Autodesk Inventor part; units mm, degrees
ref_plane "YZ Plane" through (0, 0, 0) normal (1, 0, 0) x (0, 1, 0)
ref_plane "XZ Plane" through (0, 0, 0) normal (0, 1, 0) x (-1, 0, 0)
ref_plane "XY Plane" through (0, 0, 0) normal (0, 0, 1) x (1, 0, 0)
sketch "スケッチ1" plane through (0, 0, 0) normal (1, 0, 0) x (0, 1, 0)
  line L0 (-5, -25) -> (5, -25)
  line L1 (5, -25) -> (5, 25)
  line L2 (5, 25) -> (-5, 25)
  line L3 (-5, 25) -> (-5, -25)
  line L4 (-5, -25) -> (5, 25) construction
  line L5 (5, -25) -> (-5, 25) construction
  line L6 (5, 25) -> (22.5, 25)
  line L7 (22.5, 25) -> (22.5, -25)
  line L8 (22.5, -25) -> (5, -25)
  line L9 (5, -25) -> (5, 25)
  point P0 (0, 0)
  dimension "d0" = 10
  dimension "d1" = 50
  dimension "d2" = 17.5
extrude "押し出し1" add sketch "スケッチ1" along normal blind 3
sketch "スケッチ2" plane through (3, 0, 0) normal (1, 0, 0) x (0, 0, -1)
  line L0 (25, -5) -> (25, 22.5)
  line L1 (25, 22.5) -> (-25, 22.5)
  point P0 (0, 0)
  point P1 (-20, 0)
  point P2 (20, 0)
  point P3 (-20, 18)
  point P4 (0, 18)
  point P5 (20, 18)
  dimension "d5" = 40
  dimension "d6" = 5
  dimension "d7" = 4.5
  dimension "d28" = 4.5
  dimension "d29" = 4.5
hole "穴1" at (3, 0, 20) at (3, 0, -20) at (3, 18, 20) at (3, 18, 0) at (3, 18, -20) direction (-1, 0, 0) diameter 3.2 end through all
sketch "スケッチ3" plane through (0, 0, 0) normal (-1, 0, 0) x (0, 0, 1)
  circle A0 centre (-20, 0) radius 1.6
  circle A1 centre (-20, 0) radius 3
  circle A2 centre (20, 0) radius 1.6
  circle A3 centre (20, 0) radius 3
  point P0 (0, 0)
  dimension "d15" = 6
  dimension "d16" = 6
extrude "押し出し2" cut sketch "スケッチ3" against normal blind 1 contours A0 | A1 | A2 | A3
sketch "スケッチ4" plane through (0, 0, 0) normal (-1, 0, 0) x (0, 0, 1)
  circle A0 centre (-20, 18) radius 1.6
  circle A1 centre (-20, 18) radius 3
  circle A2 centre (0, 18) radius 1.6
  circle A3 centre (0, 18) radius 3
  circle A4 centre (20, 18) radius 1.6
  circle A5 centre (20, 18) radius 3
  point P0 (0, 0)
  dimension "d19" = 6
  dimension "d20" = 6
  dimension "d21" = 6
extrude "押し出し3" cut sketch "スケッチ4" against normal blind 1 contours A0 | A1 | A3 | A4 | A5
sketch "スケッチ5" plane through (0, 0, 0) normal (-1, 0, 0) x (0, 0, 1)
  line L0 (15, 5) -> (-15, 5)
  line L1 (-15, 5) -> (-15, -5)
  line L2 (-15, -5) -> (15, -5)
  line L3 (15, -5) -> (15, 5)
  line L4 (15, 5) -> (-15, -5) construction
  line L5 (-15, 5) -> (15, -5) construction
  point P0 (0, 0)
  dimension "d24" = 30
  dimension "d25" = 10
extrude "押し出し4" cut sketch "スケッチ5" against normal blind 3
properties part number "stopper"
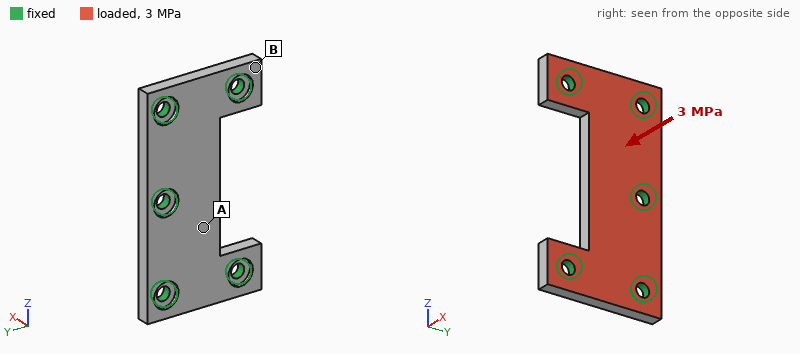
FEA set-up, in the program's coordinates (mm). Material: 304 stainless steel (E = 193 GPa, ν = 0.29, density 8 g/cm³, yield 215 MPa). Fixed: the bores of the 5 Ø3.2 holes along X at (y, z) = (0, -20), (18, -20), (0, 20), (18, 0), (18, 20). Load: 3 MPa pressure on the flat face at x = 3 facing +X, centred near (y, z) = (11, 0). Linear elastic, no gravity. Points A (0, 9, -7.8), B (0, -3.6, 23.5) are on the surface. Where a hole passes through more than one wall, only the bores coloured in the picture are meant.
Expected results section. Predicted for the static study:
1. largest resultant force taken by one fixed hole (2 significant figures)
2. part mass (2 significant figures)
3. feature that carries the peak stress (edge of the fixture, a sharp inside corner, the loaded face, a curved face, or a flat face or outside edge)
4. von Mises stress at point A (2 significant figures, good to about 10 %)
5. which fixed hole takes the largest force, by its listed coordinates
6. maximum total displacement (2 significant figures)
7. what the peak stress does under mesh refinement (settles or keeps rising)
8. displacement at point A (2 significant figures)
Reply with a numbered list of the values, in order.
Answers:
1. 980 N
2. 24 g
3. edge of the fixture
4. 62 MPa
5. (18, 0)
6. 23 µm
7. keeps rising
8. 14 µm
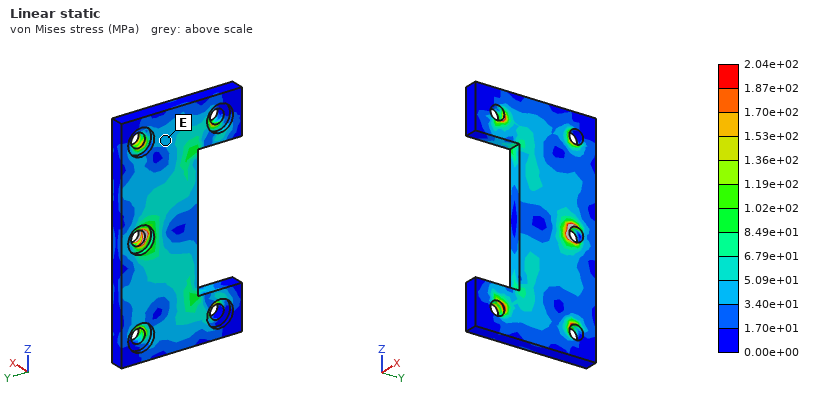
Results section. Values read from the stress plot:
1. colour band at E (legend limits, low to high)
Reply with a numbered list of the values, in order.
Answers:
1. 3.40e+01 to 5.09e+01 MPa
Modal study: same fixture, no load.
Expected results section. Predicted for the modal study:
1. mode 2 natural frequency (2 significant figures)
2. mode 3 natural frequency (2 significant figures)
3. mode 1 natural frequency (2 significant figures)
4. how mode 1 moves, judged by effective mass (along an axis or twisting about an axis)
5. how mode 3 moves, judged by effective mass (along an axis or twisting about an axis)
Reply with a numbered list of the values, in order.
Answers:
1. 24 kHz
2. 33 kHz
3. 16 kHz
4. along X
5. along X
